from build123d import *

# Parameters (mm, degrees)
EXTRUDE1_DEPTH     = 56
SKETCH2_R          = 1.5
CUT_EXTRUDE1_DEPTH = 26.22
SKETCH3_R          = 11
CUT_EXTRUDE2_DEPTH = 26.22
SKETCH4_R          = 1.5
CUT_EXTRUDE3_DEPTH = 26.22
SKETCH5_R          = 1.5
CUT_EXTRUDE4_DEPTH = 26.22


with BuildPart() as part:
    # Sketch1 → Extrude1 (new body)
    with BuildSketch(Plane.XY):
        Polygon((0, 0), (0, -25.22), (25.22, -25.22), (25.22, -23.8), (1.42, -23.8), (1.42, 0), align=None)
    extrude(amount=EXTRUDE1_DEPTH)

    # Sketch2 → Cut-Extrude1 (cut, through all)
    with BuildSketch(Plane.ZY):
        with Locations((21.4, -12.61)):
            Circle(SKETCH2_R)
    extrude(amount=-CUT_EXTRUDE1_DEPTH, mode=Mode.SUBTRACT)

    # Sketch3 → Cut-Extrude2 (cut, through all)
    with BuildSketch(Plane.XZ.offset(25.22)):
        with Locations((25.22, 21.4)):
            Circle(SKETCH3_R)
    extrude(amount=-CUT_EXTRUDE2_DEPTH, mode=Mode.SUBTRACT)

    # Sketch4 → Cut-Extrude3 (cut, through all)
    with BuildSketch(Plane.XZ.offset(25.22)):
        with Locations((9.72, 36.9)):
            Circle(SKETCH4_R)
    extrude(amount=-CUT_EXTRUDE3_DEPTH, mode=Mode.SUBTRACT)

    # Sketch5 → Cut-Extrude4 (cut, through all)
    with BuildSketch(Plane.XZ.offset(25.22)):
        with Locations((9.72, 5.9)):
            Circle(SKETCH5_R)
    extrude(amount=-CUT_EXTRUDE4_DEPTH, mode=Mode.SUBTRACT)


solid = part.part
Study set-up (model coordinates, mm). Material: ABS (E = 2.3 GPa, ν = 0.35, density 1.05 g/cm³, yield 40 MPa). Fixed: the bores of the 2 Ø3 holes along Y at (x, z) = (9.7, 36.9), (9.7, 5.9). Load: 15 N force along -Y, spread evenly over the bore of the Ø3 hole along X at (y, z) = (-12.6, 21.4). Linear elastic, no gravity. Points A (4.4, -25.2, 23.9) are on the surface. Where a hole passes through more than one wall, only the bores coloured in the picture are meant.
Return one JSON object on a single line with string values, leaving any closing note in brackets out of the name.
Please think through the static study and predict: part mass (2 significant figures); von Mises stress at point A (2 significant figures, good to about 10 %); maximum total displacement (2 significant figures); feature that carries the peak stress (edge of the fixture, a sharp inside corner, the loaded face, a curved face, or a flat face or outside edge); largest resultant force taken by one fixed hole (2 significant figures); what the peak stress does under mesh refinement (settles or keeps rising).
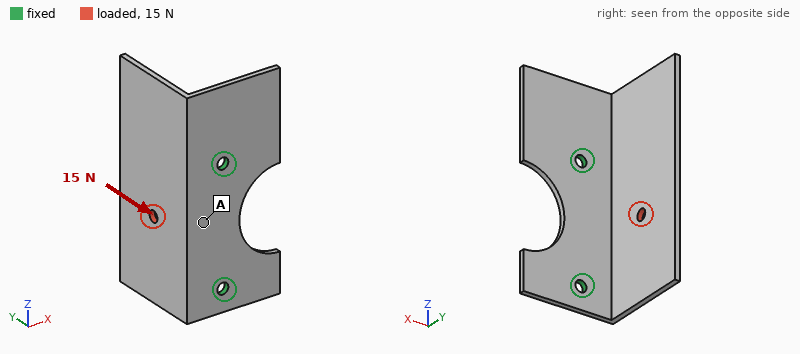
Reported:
{"part mass": "3.8 g", "von Mises stress at point A": "1.7 MPa", "maximum total displacement": "0.66 mm", "feature that carries the peak stress": "edge of the fixture", "largest resultant force taken by one fixed hole": "7.6 N", "what the peak stress does under mesh refinement": "keeps rising"}
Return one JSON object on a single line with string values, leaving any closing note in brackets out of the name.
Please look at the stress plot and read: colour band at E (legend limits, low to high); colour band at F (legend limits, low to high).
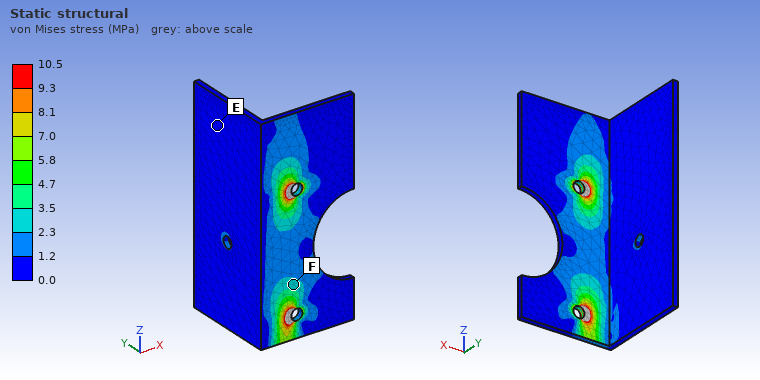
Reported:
{"colour band at E": "0.0 to 1.2 MPa", "colour band at F": "2.3 to 3.5 MPa"}
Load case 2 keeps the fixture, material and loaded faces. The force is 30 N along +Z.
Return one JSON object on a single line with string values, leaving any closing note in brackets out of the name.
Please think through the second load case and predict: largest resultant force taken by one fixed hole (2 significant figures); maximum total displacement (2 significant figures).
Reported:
{"largest resultant force taken by one fixed hole": "21 N", "maximum total displacement": "0.62 mm"}
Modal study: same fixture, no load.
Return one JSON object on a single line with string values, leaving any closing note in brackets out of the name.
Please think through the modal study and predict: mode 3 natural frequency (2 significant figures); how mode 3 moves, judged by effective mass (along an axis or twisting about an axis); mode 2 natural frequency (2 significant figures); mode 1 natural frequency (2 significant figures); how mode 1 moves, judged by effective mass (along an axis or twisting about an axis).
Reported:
{"mode 3 natural frequency": "960 Hz", "how mode 3 moves, judged by effective mass": "along Y", "mode 2 natural frequency": "590 Hz", "mode 1 natural frequency": "350 Hz", "how mode 1 moves, judged by effective mass": "along X"}
